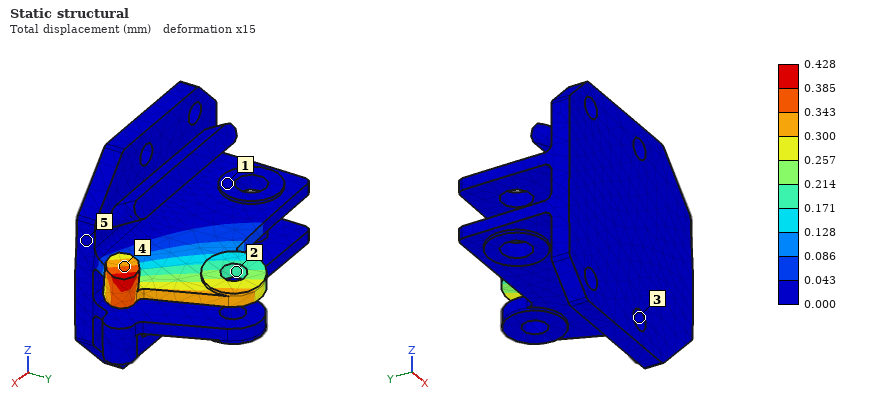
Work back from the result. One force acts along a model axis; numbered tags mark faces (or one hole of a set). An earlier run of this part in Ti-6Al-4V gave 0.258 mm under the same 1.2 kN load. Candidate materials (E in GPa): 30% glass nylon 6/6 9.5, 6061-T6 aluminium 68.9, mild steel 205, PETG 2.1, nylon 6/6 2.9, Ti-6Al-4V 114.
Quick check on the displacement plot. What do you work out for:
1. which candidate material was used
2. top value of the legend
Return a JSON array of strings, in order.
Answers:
["6061-T6 aluminium", "0.428 mm"]
